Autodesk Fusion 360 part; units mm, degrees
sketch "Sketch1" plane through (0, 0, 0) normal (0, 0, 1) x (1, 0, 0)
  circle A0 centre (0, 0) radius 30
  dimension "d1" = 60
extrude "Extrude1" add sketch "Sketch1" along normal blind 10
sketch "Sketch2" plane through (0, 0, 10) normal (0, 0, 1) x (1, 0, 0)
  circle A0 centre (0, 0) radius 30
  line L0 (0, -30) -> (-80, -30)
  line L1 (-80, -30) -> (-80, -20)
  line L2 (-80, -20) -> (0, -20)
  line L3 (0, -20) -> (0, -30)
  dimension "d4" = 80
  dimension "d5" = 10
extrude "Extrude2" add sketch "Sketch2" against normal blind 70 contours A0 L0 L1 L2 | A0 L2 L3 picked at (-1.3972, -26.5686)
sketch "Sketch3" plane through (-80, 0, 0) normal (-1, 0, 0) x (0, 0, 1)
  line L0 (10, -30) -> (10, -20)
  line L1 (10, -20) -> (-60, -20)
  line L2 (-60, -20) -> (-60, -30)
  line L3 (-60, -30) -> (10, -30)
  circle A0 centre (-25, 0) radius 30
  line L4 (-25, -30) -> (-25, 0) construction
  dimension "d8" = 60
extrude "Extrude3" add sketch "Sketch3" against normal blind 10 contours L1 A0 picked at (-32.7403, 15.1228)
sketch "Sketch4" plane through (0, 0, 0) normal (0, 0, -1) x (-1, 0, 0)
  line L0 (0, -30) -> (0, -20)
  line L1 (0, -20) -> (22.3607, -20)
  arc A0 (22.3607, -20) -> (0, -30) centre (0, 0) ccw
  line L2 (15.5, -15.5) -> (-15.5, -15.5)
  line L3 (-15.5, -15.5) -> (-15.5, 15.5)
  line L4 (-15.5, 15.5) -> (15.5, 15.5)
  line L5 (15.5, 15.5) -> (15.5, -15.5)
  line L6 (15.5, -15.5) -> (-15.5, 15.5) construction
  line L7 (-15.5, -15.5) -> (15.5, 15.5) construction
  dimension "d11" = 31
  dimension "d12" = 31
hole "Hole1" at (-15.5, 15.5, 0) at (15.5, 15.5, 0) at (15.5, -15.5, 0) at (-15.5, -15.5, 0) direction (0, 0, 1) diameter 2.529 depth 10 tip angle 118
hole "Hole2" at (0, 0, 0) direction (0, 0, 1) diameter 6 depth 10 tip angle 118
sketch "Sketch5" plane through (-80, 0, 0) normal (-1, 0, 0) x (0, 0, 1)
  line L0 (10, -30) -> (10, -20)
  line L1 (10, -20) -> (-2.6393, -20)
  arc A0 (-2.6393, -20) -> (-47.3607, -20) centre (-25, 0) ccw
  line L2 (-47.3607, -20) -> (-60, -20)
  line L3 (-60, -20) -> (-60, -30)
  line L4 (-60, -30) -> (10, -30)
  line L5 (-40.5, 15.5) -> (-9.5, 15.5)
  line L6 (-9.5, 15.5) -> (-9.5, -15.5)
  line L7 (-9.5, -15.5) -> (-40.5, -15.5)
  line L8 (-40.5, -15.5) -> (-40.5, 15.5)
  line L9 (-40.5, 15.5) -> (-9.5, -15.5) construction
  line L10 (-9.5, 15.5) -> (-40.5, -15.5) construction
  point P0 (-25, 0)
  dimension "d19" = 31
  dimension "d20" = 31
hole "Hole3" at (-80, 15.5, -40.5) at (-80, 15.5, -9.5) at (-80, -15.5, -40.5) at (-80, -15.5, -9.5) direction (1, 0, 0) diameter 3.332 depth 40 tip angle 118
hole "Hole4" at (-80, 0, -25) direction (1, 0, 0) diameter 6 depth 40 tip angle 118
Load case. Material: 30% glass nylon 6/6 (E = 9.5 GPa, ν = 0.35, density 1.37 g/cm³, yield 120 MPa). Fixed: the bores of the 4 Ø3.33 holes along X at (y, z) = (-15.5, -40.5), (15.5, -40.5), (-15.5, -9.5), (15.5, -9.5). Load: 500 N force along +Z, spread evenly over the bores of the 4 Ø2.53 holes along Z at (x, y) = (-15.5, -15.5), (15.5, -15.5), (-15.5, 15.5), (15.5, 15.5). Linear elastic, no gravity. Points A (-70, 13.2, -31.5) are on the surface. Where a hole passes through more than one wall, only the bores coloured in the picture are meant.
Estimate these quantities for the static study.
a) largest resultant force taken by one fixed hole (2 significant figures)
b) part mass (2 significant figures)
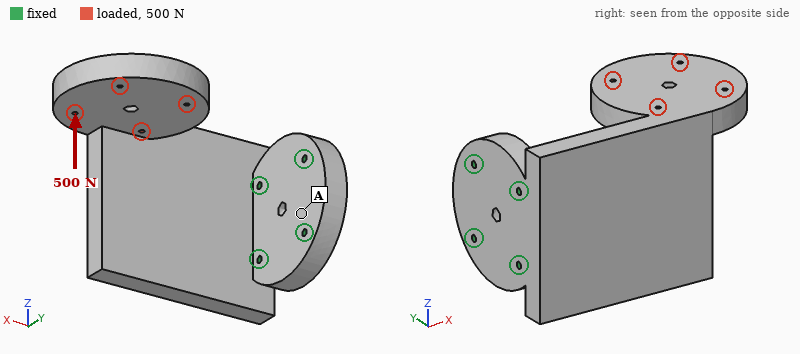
1.1 kN
150 g
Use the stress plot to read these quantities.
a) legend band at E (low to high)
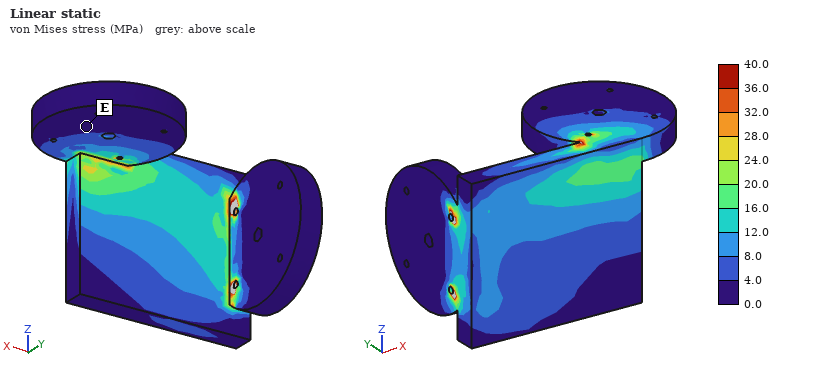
0.0 to 4.0 MPa
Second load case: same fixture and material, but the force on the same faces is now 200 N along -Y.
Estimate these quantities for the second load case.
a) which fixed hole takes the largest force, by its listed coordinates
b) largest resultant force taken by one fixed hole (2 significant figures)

(-15.5, -9.5)
250 N
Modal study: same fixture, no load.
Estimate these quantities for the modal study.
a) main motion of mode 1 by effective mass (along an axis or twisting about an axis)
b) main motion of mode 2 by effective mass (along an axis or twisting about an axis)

along Y
along Z
